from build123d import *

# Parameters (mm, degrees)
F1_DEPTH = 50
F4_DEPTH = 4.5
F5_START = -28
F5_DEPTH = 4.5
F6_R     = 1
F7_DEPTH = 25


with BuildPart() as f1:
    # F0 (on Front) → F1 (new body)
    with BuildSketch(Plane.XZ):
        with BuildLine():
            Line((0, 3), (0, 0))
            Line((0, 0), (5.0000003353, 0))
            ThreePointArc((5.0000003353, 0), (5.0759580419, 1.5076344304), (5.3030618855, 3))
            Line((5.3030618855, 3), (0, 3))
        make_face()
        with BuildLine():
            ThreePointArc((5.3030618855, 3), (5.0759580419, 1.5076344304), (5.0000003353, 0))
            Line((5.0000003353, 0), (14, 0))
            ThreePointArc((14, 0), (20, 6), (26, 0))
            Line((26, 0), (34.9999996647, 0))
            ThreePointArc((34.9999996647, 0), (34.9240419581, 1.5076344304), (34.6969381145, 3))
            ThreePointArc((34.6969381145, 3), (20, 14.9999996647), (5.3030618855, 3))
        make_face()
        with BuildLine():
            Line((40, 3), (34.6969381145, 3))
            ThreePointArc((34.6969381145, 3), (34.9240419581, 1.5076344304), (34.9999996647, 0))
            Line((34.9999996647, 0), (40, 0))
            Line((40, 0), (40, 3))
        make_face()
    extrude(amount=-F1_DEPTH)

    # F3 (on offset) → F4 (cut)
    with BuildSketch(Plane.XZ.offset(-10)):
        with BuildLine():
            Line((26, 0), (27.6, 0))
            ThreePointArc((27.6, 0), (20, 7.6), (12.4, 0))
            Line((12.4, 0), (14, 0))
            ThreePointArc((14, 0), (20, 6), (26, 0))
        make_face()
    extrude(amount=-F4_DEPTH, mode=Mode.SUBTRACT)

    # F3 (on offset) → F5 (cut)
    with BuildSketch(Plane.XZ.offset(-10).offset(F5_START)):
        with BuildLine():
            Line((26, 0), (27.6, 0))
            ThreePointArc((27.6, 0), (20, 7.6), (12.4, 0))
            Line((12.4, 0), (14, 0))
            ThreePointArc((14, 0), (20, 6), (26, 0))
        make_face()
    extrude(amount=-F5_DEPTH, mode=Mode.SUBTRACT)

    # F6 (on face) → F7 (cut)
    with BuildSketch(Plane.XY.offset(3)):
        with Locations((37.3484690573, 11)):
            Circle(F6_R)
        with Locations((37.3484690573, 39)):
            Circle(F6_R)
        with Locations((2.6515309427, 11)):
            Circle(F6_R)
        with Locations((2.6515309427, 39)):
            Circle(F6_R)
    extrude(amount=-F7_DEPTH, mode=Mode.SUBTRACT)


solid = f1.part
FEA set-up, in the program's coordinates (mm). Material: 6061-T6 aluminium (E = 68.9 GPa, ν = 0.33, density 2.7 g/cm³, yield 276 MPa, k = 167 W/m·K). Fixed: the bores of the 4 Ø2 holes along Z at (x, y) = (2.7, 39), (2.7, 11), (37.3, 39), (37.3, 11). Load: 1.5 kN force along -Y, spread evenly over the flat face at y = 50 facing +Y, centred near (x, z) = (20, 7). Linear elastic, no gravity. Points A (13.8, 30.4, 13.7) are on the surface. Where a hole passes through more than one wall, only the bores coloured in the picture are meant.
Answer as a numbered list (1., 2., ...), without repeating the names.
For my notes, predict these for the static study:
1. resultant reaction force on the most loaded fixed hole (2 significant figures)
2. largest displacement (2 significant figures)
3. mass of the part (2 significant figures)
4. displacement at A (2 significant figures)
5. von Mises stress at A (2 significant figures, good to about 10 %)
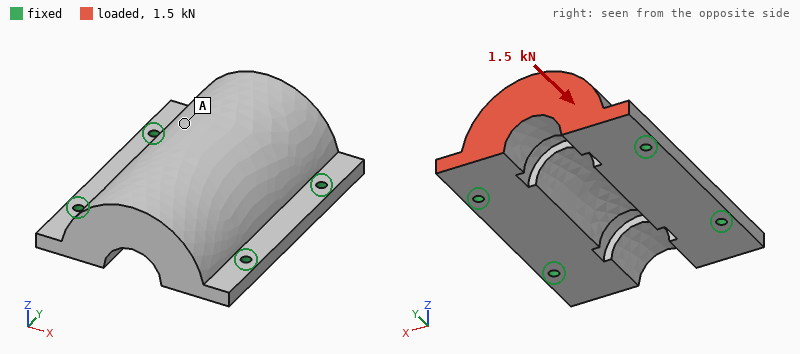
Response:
1. 480 N
2. 8.1 µm
3. 43 g
4. 4.3 µm
5. 5.0 MPa
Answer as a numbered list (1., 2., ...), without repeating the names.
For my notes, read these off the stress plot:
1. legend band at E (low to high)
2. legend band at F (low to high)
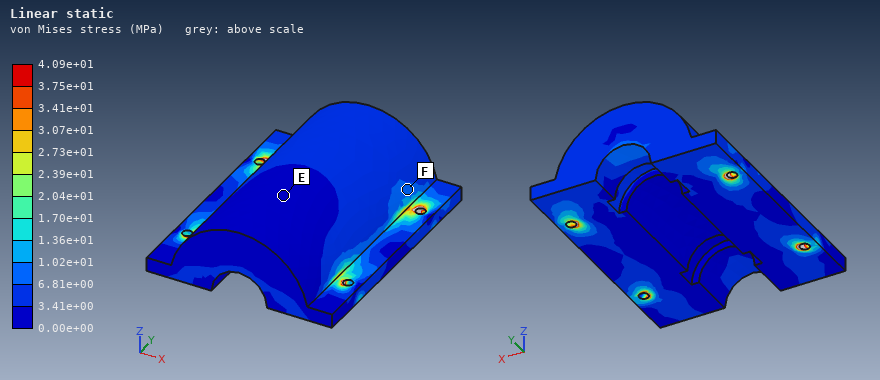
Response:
1. 0.00e+00 to 3.41e+00 MPa
2. 6.81e+00 to 1.02e+01 MPa
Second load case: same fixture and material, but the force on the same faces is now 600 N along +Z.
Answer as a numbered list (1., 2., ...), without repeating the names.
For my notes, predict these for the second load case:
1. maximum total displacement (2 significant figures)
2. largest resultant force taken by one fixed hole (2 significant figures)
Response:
1. 14 µm
2. 510 N
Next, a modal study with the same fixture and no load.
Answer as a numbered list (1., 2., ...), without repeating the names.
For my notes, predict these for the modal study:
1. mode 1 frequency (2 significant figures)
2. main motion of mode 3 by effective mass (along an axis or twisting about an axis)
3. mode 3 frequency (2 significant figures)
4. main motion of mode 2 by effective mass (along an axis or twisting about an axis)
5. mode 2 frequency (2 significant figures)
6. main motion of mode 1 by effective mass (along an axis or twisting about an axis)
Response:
1. 11 kHz
2. along X
3. 19 kHz
4. along Z
5. 13 kHz
6. along Y
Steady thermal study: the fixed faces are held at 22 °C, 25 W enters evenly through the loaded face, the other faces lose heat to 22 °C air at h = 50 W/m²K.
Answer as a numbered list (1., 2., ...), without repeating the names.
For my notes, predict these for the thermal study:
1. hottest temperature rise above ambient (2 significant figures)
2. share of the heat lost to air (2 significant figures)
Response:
1. 13 K
2. 5.6 %
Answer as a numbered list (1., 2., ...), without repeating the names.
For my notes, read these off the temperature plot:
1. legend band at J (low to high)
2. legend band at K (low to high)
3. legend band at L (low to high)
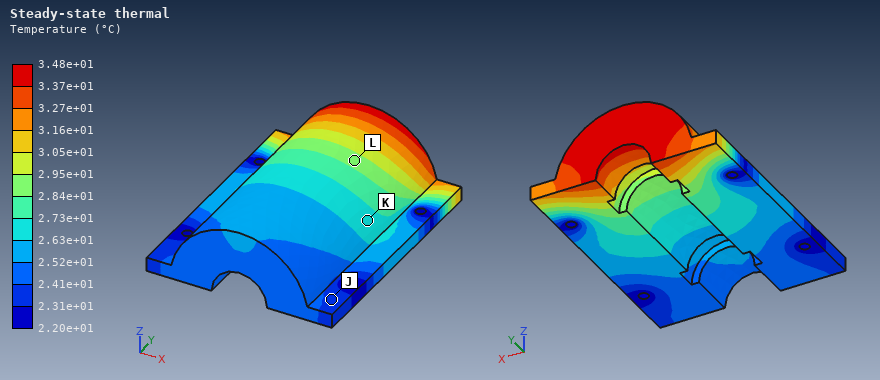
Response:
1. 2.31e+01 to 2.41e+01 °C
2. 2.63e+01 to 2.73e+01 °C
3. 2.84e+01 to 2.95e+01 °C
